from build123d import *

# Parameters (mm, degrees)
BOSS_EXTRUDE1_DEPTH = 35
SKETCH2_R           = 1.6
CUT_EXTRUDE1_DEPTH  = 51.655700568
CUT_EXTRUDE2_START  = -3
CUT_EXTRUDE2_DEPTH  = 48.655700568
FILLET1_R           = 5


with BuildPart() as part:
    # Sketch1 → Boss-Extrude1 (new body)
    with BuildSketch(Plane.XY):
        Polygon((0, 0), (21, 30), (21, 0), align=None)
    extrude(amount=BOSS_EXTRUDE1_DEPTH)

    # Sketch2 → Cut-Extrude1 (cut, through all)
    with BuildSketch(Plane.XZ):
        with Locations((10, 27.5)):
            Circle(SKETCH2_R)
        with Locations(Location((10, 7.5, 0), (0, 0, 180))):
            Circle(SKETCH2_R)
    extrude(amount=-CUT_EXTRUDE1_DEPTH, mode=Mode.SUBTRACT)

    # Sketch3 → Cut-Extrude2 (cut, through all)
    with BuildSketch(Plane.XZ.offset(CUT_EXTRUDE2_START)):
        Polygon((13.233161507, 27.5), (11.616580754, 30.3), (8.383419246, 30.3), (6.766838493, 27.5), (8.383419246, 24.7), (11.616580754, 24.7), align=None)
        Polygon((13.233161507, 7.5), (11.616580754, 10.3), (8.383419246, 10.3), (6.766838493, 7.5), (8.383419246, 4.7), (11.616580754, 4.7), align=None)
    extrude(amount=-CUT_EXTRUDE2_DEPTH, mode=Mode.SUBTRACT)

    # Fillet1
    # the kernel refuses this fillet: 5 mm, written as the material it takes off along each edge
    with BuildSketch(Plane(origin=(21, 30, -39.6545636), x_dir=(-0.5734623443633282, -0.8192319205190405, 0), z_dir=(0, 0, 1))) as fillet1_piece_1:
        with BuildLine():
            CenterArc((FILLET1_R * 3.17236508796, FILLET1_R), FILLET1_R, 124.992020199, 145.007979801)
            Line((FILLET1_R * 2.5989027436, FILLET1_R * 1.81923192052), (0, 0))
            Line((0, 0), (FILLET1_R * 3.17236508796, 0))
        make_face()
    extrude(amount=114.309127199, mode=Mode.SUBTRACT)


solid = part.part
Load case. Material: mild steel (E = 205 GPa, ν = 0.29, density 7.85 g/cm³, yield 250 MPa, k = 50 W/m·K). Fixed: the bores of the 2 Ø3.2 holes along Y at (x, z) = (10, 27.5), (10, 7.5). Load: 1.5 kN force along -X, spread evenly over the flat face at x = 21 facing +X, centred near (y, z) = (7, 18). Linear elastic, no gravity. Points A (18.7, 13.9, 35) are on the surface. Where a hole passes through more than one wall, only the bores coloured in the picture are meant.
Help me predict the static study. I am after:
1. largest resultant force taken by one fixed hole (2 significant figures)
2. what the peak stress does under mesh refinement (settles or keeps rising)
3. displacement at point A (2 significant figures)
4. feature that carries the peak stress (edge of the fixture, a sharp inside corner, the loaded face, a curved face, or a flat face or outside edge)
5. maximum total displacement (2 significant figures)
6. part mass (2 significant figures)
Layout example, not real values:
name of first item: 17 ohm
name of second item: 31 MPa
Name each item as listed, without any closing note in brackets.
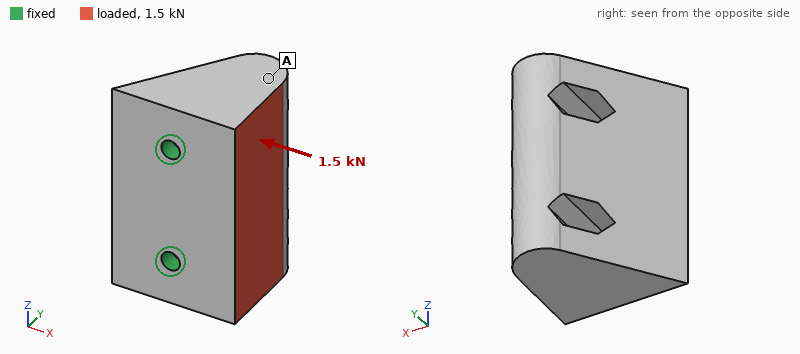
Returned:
largest resultant force taken by one fixed hole: 750 N
what the peak stress does under mesh refinement: keeps rising
displacement at point A: 12 µm
feature that carries the peak stress: edge of the fixture
maximum total displacement: 15 µm
part mass: 68 g
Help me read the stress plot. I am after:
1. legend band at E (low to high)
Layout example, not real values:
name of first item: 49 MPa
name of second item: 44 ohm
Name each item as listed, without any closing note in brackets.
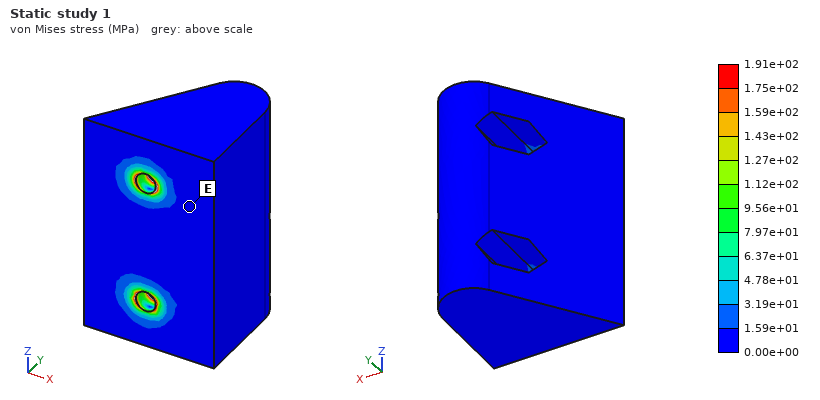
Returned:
legend band at E: 0.00e+00 to 1.59e+01 MPa
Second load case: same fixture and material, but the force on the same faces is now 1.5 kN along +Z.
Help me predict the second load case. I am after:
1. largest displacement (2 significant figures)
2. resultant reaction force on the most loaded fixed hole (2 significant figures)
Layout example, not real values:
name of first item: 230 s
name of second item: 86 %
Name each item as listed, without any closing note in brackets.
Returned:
largest displacement: 3.1 µm
resultant reaction force on the most loaded fixed hole: 1.1 kN
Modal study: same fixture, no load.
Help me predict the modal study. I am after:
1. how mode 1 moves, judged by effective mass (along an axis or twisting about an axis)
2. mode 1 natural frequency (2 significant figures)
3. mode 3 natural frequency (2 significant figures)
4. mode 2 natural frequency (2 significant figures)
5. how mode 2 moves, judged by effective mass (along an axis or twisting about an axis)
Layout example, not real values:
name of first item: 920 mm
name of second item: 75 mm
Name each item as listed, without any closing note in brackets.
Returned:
how mode 1 moves, judged by effective mass: along X
mode 1 natural frequency: 6300 Hz
mode 3 natural frequency: 21 kHz
mode 2 natural frequency: 18 kHz
how mode 2 moves, judged by effective mass: along Z
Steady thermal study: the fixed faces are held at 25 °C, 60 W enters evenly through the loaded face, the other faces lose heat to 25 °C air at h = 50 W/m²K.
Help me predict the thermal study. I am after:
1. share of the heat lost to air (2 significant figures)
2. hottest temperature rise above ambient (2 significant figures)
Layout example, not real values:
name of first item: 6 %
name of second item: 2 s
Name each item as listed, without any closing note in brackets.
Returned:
share of the heat lost to air: 9.3 %
hottest temperature rise above ambient: 63 K
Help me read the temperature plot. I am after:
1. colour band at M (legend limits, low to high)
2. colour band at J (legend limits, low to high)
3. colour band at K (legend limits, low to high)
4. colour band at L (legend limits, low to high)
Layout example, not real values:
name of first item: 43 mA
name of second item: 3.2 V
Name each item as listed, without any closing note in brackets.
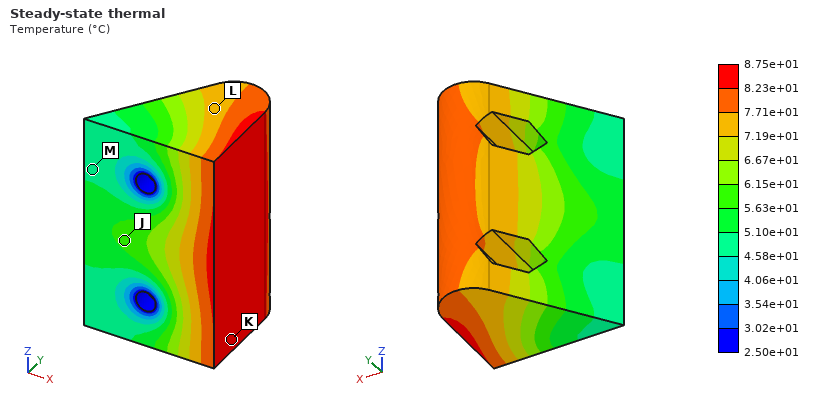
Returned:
colour band at M: 4.58e+01 to 5.10e+01 °C
colour band at J: 5.63e+01 to 6.15e+01 °C
colour band at K: 8.23e+01 to 8.75e+01 °C
colour band at L: 7.19e+01 to 7.71e+01 °C
